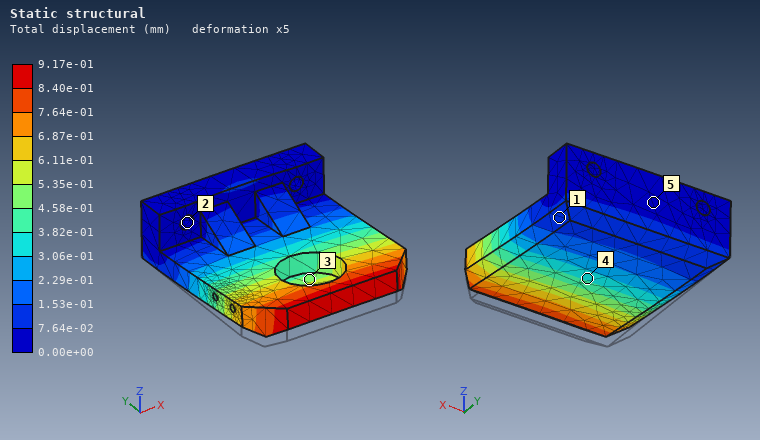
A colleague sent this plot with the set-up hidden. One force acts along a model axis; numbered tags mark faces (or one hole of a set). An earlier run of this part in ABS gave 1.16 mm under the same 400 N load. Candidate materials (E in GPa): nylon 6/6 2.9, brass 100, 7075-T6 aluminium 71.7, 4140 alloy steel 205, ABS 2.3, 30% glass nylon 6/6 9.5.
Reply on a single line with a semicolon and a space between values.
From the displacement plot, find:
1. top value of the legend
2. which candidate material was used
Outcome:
9.17e-01 mm; nylon 6/6
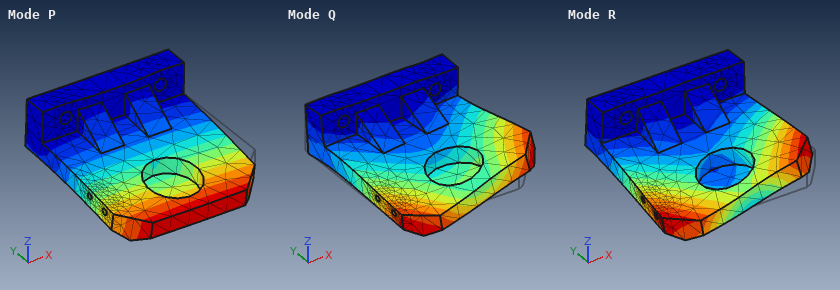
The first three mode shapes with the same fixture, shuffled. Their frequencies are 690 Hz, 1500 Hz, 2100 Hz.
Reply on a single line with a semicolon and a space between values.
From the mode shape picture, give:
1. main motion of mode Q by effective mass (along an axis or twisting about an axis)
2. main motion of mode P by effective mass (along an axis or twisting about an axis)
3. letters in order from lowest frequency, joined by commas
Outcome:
along X; along Z; P, R, Q
